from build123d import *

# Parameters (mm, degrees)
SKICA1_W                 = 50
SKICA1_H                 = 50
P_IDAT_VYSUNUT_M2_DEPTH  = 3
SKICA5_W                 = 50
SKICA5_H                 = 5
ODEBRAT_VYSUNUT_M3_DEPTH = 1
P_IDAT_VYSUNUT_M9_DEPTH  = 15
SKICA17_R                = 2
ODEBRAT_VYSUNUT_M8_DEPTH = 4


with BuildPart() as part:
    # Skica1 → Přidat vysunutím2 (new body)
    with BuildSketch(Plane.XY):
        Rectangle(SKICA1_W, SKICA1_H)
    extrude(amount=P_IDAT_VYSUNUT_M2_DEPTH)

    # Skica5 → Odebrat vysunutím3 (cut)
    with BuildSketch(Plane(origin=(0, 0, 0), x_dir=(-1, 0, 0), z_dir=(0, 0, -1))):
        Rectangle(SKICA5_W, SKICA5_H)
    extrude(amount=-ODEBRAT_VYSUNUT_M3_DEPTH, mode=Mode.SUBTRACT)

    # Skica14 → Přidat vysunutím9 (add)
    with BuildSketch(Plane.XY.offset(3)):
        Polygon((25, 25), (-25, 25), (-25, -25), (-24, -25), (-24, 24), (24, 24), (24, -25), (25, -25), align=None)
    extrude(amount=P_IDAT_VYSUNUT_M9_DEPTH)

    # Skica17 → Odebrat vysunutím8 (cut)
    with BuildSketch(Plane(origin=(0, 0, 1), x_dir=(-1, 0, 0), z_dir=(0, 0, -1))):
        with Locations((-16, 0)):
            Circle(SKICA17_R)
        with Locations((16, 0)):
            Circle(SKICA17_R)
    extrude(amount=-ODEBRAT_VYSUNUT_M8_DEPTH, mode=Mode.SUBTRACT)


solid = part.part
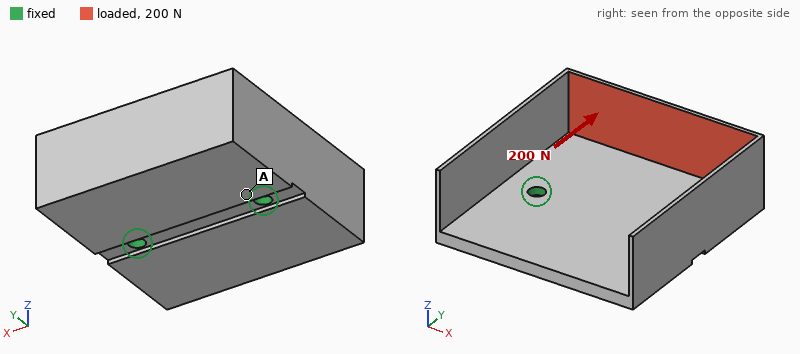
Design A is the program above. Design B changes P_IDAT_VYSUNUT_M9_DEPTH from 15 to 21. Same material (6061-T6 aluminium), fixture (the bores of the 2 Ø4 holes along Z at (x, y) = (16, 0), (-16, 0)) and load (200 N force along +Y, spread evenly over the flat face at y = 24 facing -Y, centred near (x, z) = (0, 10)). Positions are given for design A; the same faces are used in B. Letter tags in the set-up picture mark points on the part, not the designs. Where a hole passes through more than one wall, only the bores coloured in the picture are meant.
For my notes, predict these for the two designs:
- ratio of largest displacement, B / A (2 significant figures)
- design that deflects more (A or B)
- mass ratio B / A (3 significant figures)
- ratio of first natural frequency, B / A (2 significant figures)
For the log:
1.7
B
1.09
0.87
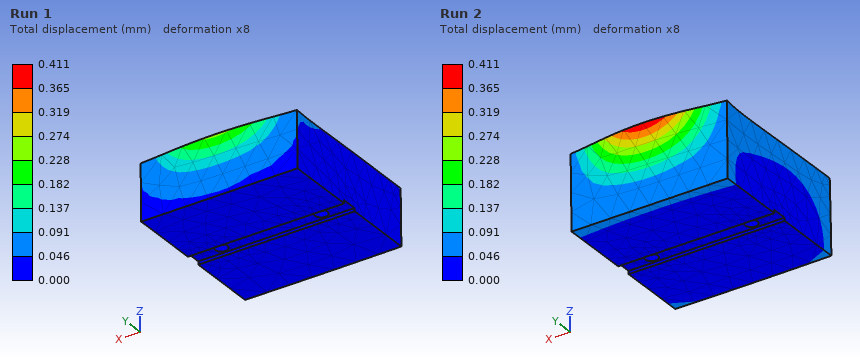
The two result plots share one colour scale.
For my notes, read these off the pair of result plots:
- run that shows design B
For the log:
Run 2
